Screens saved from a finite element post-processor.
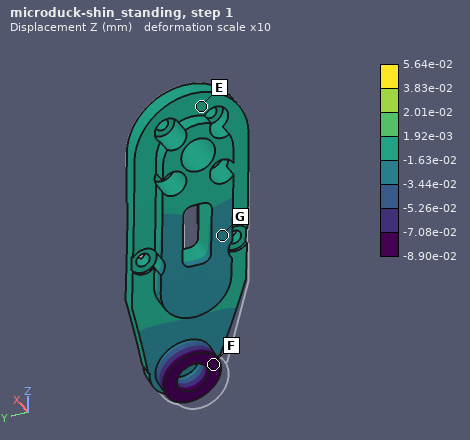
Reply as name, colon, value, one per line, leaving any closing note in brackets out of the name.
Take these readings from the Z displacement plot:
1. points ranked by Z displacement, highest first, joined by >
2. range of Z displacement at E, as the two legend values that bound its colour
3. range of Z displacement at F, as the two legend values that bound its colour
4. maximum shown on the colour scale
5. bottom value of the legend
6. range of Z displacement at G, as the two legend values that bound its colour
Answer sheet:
points ranked by Z displacement, highest first, joined by >: E > G > F
range of Z displacement at E, as the two legend values that bound its colour: -1.63e-02 to 1.92e-03 mm
range of Z displacement at F, as the two legend values that bound its colour: -8.90e-02 to -7.08e-02 mm
maximum shown on the colour scale: 5.64e-02 mm
bottom value of the legend: -8.90e-02 mm
range of Z displacement at G, as the two legend values that bound its colour: -3.44e-02 to -1.63e-02 mm
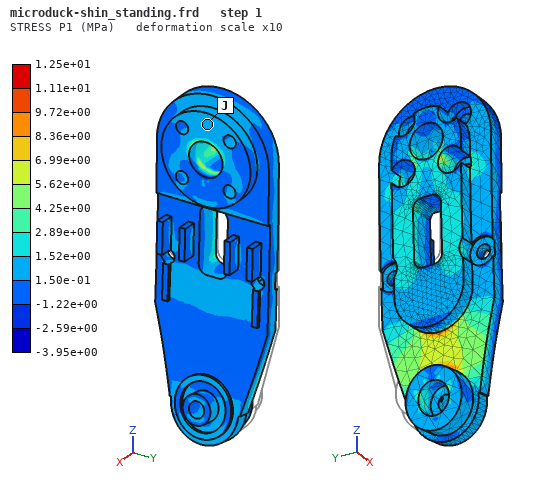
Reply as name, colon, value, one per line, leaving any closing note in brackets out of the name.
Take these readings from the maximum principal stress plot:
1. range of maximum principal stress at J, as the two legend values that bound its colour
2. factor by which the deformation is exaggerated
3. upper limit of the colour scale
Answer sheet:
range of maximum principal stress at J, as the two legend values that bound its colour: 1.50e-01 to 1.52e+00 MPa
factor by which the deformation is exaggerated: 10
upper limit of the colour scale: 1.25e+01 MPa
